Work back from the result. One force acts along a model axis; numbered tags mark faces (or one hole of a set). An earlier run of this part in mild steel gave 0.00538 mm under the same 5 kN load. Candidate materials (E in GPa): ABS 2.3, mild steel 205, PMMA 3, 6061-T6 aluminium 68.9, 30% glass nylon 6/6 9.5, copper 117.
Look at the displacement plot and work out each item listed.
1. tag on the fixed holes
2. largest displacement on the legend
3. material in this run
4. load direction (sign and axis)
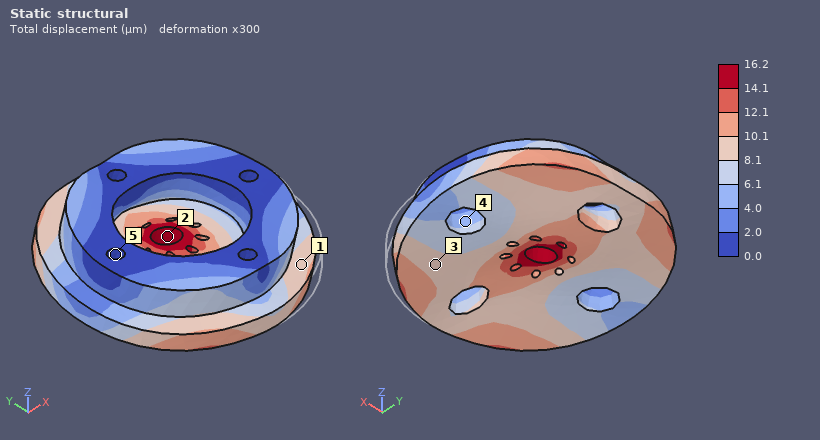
5
16.2 µm
6061-T6 aluminium
+Y
